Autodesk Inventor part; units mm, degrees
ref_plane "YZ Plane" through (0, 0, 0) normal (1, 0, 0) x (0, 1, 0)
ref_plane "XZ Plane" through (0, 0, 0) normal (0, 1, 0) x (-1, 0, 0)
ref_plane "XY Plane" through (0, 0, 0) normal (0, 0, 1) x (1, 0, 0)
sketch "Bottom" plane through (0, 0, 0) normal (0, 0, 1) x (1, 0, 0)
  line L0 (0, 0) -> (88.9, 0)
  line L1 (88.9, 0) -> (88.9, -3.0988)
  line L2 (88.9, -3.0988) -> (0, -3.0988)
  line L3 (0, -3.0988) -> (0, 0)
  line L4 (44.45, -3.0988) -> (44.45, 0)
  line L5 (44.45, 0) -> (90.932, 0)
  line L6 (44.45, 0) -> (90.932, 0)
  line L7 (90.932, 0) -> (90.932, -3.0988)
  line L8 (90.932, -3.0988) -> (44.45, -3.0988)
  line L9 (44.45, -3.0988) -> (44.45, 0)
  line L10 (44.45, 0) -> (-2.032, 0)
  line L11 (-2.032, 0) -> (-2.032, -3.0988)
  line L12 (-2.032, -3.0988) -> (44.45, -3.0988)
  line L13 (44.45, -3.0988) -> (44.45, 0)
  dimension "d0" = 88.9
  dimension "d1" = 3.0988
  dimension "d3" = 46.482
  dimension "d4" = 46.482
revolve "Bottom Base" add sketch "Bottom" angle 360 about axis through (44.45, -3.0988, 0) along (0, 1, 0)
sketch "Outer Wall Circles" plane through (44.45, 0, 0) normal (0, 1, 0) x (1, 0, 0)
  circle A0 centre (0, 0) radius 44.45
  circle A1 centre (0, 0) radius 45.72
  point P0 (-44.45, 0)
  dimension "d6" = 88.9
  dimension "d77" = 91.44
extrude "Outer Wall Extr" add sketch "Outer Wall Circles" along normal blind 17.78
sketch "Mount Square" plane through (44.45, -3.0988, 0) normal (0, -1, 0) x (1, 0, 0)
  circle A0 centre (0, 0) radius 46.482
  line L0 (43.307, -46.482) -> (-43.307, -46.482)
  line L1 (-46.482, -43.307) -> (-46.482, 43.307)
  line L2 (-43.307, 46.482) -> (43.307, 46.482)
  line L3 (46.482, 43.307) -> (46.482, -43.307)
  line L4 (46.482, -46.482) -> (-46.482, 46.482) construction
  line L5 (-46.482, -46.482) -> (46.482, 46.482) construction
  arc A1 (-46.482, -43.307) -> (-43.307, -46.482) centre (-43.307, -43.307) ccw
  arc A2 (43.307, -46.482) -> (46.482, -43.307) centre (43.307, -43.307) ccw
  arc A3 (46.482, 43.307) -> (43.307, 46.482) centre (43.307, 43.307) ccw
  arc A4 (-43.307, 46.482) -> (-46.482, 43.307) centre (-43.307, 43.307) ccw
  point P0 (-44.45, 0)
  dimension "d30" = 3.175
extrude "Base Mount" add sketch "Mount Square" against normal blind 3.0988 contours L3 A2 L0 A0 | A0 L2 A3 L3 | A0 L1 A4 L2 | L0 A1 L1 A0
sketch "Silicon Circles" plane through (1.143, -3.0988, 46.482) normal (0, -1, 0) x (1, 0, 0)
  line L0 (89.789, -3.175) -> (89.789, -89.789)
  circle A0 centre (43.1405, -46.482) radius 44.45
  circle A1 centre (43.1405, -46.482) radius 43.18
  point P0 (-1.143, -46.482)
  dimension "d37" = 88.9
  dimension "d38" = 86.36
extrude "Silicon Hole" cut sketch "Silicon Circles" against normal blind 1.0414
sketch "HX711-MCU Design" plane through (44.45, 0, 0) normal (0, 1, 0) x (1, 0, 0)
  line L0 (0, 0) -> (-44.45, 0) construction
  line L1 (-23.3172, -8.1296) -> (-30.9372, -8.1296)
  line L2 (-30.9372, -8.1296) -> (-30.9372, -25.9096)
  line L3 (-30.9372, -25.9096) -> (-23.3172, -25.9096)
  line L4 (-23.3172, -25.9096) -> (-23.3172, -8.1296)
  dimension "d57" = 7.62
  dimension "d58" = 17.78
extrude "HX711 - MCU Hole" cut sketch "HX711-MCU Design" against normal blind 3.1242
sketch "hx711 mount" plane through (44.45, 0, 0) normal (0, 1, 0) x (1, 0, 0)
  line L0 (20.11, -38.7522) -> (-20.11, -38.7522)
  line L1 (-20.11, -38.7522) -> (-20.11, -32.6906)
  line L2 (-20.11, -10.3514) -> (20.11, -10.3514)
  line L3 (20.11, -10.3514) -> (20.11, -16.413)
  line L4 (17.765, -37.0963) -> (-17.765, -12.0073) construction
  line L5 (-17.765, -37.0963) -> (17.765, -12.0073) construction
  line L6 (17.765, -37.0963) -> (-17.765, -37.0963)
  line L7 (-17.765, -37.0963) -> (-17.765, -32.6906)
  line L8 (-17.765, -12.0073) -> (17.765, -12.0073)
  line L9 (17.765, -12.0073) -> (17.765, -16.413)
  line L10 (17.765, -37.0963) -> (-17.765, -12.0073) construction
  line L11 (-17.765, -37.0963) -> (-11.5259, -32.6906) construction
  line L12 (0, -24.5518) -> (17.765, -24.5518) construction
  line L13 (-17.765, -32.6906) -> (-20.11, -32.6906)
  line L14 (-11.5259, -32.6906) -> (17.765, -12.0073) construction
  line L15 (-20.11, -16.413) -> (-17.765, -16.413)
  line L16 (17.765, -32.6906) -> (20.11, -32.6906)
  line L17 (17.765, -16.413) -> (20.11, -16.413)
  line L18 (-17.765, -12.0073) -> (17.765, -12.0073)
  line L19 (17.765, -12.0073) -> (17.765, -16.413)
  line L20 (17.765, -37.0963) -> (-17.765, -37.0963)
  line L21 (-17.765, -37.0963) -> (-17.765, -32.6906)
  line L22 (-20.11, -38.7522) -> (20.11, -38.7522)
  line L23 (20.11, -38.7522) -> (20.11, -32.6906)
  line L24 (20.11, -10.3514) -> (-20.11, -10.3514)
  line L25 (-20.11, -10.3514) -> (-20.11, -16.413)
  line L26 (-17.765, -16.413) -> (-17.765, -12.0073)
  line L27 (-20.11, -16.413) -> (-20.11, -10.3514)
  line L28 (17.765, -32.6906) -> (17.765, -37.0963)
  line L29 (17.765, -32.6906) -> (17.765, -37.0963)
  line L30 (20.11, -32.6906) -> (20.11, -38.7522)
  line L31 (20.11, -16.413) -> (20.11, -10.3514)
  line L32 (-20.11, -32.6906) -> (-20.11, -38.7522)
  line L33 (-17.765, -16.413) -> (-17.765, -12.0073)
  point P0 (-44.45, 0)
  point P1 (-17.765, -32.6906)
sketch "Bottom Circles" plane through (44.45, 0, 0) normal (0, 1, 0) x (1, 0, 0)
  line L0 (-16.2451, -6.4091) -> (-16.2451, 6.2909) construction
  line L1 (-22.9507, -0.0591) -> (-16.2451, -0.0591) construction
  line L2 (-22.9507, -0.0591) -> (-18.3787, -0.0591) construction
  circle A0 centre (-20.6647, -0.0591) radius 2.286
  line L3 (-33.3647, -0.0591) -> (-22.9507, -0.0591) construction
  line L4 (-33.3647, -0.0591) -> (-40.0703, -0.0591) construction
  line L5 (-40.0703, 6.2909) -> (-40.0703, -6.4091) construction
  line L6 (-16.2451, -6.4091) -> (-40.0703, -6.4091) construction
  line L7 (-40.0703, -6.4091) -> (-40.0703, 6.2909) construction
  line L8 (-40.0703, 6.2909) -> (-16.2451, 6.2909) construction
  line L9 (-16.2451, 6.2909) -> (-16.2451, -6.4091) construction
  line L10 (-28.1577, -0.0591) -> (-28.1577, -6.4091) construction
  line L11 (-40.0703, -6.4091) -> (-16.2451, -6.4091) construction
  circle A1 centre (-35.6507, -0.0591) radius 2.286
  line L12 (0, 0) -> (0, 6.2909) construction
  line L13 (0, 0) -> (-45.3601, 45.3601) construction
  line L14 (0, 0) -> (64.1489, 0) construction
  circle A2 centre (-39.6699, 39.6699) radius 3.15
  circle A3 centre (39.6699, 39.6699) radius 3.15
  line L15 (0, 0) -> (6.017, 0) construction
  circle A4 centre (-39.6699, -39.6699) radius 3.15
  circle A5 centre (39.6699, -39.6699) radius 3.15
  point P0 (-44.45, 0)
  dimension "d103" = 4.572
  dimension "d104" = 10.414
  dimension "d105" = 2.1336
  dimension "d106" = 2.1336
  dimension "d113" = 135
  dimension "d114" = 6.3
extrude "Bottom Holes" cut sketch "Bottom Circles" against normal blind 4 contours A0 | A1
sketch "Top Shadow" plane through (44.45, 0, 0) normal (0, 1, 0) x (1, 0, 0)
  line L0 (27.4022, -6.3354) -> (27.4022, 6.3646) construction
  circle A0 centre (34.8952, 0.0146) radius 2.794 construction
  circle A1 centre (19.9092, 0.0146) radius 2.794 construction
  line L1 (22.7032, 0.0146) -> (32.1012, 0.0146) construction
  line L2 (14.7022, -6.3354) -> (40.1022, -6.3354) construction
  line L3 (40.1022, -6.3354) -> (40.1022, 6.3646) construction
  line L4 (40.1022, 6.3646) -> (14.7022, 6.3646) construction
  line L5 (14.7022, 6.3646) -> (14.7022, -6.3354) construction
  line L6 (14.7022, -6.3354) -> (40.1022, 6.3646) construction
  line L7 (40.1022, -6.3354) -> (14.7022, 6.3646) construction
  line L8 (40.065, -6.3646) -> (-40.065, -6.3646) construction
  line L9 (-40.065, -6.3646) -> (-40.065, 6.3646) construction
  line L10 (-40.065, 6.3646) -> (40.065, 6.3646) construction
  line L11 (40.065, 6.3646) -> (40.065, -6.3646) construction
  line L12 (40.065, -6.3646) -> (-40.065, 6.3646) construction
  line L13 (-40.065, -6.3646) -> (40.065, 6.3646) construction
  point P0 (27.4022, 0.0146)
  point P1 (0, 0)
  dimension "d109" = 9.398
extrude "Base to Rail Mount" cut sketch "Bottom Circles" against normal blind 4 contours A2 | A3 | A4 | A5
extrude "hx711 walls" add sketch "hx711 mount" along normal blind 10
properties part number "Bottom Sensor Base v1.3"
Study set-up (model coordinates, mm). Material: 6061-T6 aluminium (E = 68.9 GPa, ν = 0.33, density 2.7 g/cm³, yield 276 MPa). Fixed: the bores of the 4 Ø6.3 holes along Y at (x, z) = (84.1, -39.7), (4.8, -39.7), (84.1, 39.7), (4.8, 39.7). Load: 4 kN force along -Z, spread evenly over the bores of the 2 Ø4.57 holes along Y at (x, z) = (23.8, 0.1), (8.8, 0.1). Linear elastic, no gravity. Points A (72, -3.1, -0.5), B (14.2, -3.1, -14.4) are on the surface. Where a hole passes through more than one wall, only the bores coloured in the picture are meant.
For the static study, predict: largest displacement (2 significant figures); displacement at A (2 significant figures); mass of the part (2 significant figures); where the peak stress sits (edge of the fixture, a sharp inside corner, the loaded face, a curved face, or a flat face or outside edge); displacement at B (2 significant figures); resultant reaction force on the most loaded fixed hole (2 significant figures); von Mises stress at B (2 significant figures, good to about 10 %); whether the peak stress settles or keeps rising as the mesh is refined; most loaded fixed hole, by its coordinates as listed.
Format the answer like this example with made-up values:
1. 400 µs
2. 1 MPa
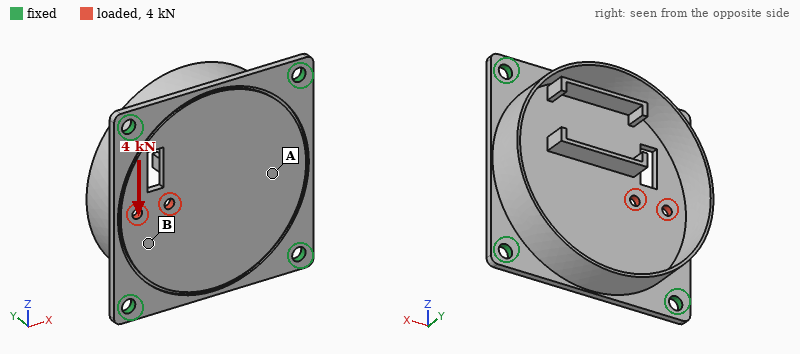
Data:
1. 18 µm
2. 3.3 µm
3. 91 g
4. edge of the fixture
5. 12 µm
6. 1.7 kN
7. 22 MPa
8. keeps rising
9. (4.8, -39.7)
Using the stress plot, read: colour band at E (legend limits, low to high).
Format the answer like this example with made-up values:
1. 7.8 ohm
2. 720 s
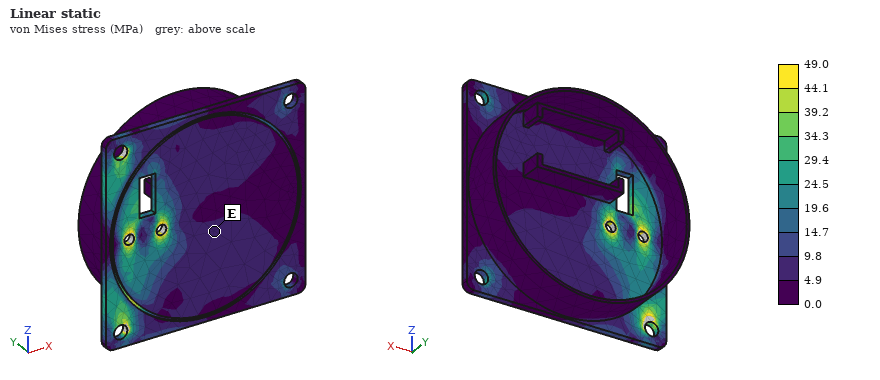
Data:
1. 4.9 to 9.8 MPa
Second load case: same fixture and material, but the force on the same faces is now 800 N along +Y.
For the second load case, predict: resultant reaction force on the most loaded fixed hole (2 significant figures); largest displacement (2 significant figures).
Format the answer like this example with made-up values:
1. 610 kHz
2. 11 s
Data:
1. 410 N
2. 0.23 mm
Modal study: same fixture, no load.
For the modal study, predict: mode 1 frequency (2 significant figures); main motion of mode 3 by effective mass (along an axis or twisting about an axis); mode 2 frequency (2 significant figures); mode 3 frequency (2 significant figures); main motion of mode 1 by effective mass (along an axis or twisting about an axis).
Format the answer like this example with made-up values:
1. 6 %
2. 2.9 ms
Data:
1. 2100 Hz
2. twisting about Z
3. 3000 Hz
4. 3200 Hz
5. along Y
